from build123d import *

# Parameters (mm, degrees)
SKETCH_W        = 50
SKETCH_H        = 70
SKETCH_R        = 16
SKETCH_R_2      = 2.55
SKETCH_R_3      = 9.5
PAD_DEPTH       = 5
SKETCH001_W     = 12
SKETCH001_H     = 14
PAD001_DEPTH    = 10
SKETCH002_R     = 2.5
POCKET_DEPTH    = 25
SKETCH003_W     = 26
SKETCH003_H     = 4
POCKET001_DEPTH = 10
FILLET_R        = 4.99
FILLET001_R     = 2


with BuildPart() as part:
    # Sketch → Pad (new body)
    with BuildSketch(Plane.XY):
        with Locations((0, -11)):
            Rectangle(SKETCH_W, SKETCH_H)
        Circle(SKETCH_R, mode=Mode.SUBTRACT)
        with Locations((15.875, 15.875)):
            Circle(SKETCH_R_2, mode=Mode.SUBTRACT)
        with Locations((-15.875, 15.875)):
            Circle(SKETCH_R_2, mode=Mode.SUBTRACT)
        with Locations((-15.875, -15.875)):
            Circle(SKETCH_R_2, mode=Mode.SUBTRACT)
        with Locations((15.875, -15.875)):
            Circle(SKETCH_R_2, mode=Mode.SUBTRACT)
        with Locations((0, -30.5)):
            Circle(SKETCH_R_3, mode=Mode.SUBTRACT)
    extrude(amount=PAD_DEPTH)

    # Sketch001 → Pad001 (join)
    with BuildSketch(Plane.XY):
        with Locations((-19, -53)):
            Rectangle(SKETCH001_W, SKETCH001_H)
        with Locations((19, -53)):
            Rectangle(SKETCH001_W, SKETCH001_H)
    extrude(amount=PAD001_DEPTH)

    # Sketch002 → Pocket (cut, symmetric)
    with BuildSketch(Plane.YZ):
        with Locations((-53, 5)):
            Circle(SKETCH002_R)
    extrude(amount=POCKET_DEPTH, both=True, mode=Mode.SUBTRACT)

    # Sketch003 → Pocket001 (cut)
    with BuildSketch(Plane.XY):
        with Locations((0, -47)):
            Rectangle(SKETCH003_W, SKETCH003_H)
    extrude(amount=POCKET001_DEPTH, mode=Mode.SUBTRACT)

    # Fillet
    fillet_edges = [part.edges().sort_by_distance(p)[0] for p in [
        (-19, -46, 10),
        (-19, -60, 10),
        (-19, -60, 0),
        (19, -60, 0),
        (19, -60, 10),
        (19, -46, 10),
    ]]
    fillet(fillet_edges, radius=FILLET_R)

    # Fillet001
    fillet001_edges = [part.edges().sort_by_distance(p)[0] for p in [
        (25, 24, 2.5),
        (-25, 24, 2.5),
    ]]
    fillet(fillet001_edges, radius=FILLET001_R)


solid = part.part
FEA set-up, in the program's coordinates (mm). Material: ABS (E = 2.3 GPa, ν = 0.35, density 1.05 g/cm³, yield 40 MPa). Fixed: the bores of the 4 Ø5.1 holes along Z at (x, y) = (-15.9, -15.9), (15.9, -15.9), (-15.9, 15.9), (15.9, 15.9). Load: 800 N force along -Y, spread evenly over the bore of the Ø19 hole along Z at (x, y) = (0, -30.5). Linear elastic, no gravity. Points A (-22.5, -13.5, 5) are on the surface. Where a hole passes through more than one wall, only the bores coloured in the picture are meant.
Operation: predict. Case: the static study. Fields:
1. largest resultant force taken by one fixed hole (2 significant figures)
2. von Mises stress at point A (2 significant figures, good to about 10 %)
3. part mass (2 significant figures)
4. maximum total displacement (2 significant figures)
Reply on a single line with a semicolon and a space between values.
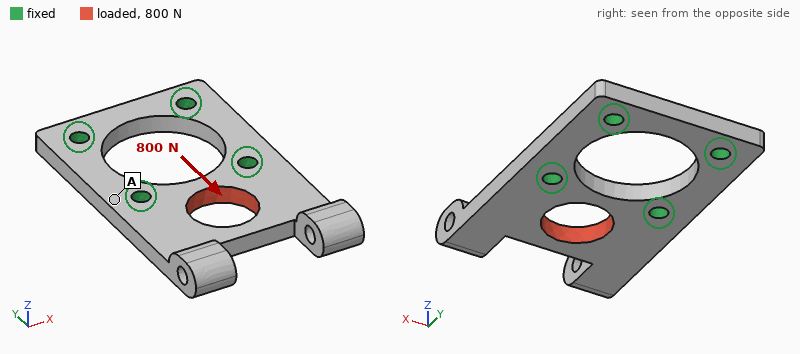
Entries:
420 N; 1.5 MPa; 15 g; 0.11 mm
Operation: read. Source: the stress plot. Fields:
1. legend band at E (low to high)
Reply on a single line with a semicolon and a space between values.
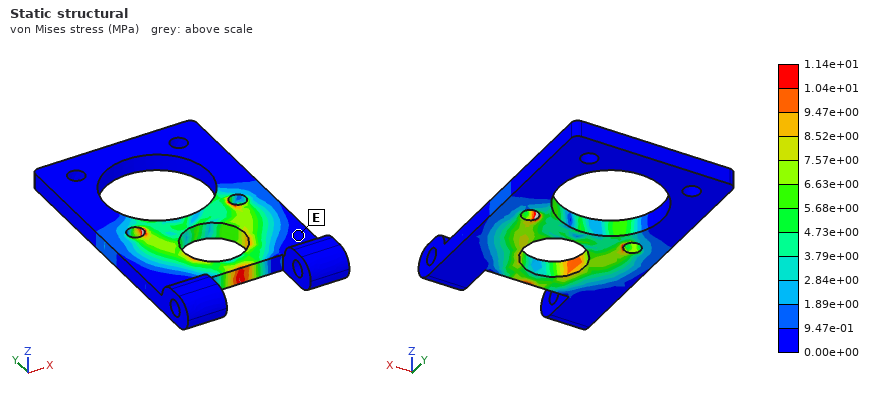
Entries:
0.00e+00 to 9.47e-01 MPa
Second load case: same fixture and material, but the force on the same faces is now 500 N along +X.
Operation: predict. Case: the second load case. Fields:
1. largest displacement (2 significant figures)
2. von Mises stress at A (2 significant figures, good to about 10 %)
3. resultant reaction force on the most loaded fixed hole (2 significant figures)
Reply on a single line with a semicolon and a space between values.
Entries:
0.26 mm; 3.5 MPa; 280 N
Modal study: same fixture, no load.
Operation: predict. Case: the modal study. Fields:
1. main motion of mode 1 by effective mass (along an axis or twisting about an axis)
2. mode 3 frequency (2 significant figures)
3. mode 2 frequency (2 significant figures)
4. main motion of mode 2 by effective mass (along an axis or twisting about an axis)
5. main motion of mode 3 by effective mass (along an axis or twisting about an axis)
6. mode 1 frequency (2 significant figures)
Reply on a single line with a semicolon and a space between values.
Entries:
along Z; 2100 Hz; 830 Hz; twisting about Y; along X; 620 Hz
